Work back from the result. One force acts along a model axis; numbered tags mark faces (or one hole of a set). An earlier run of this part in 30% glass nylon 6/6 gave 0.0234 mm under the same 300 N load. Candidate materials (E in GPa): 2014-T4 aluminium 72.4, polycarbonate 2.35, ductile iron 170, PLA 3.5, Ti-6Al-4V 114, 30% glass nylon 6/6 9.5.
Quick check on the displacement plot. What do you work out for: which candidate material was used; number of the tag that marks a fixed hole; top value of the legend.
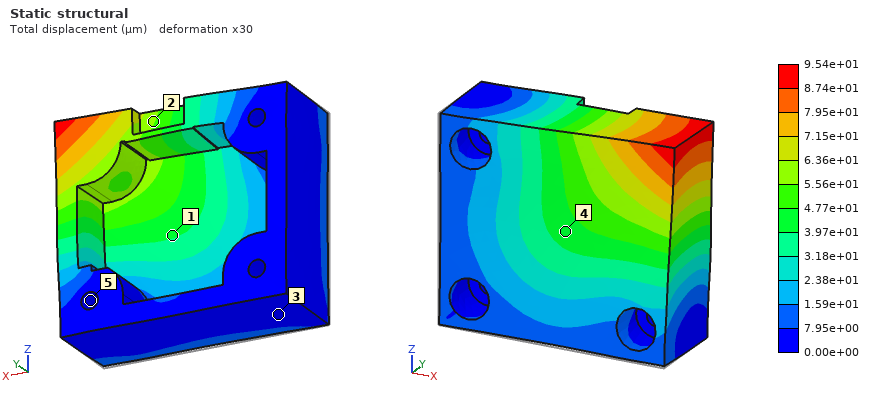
polycarbonate
5
9.54e+01 µm
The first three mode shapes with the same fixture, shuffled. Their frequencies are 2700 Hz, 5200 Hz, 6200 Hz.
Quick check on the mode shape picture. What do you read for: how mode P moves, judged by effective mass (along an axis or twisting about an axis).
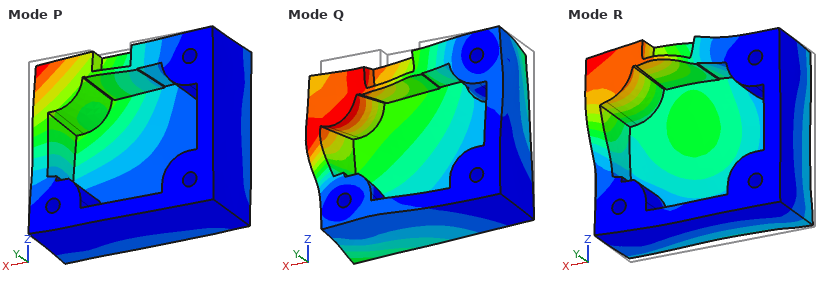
along Y
